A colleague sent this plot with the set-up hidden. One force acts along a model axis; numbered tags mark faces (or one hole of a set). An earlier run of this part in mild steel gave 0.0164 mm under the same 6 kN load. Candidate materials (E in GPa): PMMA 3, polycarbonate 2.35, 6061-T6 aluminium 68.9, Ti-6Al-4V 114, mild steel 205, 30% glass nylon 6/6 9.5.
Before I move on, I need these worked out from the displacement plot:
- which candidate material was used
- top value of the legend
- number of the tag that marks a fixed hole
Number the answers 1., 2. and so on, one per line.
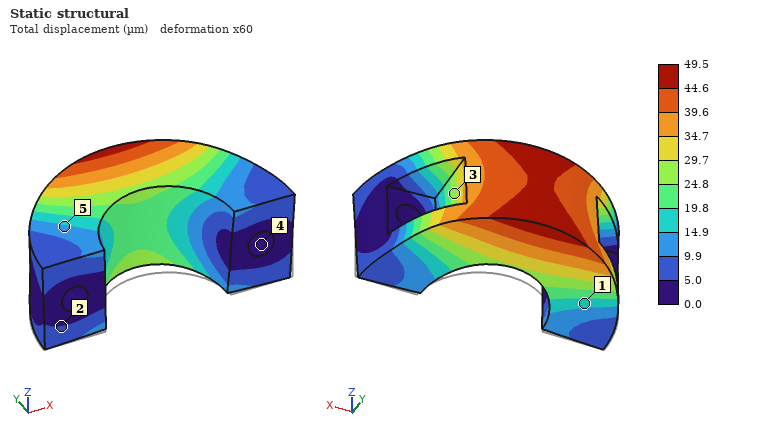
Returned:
1. 6061-T6 aluminium
2. 49.5 µm
3. 4
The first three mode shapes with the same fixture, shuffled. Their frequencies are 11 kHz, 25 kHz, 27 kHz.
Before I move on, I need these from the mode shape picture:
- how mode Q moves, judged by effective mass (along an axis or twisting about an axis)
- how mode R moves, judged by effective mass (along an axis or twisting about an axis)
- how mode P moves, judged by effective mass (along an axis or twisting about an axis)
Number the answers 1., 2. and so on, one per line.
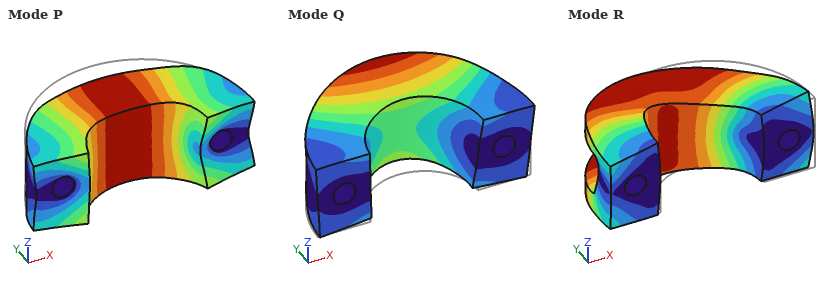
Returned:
1. along Z
2. along X
3. along Y
